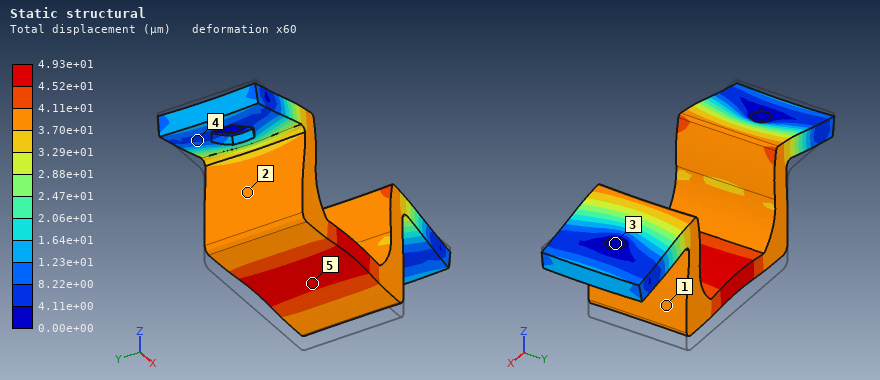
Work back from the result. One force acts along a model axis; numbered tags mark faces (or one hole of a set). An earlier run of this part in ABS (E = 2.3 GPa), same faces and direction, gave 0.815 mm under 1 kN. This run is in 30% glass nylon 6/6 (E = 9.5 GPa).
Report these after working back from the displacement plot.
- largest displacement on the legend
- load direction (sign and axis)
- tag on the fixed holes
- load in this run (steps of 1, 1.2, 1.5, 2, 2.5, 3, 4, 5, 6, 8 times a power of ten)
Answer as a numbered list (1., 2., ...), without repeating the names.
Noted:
1. 4.93e+01 µm
2. +Z
3. 3
4. 250 N
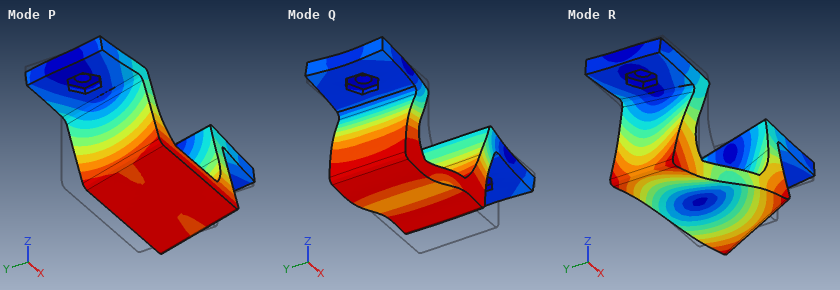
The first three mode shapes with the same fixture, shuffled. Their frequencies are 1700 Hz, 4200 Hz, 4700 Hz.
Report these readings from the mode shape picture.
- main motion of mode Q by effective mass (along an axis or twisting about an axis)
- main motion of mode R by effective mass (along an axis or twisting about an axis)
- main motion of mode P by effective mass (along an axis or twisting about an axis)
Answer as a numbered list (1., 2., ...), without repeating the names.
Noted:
1. along X
2. twisting about Z
3. along Y
